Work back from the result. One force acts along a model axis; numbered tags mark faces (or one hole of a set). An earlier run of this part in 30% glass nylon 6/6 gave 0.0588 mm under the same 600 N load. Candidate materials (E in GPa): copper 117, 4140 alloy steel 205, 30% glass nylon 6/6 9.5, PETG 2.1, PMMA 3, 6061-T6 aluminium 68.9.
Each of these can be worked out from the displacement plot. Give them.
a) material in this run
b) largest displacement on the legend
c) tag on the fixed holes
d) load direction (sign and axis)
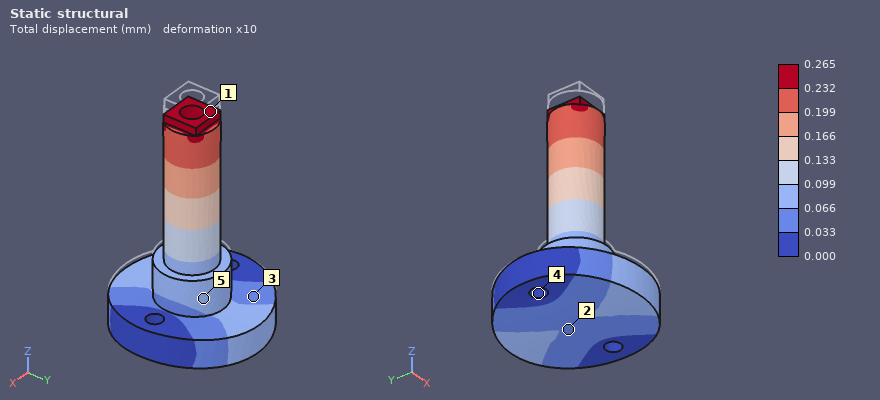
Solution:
PETG
0.265 mm
4
-Z
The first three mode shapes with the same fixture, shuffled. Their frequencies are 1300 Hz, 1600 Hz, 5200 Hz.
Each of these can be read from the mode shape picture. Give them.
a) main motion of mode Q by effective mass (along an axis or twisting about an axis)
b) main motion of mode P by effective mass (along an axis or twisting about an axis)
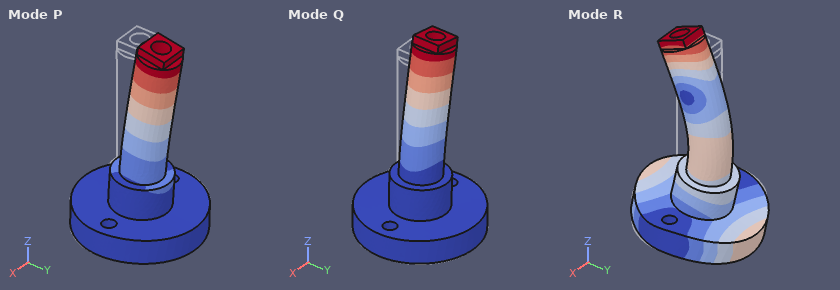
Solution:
along X
along Y
